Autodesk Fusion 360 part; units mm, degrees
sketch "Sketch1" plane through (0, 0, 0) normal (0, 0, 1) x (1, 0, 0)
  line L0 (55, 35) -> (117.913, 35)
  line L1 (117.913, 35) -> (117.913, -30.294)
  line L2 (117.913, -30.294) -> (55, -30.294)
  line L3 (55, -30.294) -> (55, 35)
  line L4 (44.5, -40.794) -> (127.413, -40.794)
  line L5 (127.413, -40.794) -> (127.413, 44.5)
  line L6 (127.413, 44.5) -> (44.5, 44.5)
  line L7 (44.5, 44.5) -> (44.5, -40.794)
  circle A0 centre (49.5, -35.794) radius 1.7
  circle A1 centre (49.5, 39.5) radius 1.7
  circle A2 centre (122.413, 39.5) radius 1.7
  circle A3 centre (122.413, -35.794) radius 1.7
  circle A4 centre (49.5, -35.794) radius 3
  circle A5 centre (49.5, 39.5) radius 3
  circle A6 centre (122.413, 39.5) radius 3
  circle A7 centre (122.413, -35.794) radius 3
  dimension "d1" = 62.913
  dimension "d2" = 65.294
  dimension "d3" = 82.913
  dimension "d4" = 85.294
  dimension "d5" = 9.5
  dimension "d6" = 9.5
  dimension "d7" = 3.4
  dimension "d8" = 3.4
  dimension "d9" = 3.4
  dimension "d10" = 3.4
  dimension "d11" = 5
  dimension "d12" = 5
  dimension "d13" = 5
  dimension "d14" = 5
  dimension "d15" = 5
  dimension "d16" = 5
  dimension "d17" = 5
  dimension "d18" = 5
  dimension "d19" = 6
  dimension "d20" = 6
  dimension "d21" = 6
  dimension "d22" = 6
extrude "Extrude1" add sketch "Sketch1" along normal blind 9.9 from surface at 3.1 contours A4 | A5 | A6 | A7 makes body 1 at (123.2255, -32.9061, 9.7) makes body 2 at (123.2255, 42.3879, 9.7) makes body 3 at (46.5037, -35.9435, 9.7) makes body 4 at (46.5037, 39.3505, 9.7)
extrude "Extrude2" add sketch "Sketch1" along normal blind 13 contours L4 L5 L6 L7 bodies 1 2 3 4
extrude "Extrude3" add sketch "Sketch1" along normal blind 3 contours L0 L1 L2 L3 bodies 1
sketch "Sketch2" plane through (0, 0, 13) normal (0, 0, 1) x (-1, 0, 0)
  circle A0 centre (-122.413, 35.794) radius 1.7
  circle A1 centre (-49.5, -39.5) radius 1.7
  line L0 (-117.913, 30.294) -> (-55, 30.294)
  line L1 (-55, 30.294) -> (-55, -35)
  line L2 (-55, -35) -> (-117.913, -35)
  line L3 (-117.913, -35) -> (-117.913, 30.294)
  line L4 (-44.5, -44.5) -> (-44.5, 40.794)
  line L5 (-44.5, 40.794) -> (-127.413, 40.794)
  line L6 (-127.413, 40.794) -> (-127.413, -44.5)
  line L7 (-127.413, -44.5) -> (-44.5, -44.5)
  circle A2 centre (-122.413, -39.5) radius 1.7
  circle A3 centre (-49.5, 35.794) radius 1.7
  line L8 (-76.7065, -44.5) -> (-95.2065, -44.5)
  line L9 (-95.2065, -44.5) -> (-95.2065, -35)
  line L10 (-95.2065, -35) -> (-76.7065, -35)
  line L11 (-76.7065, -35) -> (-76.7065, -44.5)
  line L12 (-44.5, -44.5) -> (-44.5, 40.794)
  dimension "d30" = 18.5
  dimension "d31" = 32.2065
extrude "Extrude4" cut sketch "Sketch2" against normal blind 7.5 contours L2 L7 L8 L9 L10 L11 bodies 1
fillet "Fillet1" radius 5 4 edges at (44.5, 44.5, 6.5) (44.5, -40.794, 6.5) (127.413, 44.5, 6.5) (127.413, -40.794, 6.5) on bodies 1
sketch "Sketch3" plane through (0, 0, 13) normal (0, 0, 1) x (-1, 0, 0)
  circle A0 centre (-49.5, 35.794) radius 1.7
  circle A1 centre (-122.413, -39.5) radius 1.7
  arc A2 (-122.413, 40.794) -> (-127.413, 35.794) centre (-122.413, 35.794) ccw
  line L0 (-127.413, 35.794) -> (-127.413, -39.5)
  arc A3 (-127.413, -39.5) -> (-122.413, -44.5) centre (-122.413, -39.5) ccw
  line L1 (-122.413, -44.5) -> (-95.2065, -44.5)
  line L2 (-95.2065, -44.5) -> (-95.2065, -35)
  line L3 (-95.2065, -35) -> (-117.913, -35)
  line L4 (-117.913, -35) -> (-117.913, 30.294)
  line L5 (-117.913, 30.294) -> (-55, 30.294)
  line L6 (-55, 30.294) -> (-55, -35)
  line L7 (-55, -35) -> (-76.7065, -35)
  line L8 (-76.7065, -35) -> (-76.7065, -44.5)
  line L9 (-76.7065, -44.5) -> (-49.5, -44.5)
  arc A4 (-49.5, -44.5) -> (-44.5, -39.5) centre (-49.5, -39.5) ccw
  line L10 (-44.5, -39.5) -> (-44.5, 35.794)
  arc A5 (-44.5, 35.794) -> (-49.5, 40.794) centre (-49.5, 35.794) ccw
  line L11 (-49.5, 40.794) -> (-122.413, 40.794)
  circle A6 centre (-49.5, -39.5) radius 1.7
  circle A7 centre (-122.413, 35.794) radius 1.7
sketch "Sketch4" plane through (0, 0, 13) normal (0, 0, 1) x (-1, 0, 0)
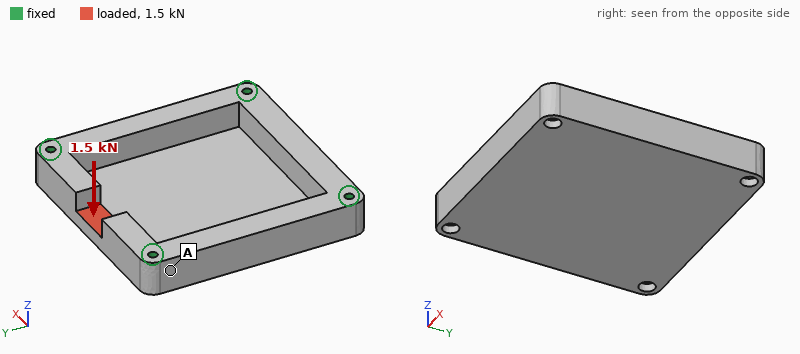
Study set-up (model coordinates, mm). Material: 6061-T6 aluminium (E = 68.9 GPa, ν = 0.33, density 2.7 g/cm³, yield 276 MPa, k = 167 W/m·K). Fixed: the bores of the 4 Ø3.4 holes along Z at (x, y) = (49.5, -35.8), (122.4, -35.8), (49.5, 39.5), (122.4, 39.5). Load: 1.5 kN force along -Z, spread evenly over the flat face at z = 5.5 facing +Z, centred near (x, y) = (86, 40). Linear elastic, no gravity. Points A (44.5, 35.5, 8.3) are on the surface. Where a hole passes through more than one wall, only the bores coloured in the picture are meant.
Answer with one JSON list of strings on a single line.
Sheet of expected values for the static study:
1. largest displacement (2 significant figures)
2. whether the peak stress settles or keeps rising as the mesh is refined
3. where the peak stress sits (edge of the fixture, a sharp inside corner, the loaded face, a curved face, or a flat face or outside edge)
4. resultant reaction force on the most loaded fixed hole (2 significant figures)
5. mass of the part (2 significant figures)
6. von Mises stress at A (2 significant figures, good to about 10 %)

["55 µm", "keeps rising", "edge of the fixture", "1.6 kN", "130 g", "13 MPa"]
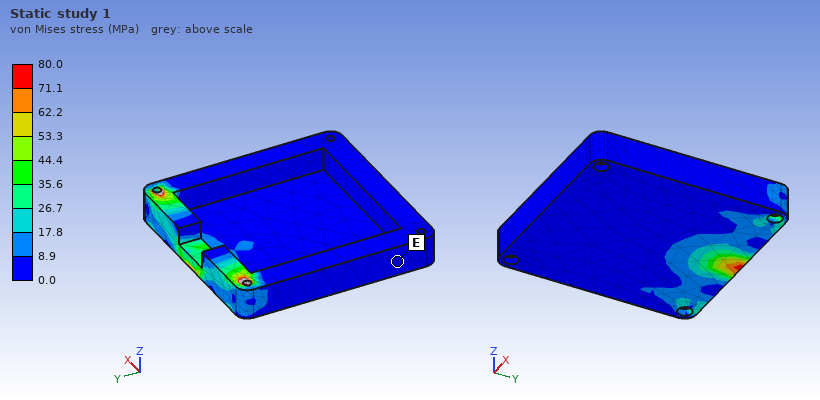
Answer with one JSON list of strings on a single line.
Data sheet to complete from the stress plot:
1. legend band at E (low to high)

["0.0 to 8.9 MPa"]
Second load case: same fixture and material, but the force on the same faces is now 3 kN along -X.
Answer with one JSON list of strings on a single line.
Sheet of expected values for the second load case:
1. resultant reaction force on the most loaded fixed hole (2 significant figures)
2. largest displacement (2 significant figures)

["1.3 kN", "15 µm"]
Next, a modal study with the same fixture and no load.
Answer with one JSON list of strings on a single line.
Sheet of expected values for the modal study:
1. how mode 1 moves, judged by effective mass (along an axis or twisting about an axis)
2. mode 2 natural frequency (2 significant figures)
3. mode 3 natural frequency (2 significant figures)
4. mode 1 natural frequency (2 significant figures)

["along Z", "7900 Hz", "8100 Hz", "4800 Hz"]
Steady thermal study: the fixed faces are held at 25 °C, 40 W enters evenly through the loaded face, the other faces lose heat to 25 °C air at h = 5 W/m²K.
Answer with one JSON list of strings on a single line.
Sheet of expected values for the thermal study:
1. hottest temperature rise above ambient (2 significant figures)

["31 K"]
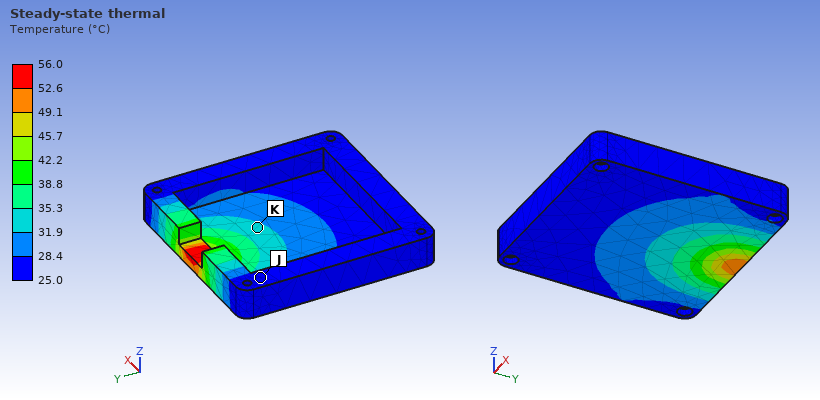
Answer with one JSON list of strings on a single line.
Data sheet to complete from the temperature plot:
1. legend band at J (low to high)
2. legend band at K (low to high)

["25.0 to 28.4 °C", "31.9 to 35.3 °C"]
